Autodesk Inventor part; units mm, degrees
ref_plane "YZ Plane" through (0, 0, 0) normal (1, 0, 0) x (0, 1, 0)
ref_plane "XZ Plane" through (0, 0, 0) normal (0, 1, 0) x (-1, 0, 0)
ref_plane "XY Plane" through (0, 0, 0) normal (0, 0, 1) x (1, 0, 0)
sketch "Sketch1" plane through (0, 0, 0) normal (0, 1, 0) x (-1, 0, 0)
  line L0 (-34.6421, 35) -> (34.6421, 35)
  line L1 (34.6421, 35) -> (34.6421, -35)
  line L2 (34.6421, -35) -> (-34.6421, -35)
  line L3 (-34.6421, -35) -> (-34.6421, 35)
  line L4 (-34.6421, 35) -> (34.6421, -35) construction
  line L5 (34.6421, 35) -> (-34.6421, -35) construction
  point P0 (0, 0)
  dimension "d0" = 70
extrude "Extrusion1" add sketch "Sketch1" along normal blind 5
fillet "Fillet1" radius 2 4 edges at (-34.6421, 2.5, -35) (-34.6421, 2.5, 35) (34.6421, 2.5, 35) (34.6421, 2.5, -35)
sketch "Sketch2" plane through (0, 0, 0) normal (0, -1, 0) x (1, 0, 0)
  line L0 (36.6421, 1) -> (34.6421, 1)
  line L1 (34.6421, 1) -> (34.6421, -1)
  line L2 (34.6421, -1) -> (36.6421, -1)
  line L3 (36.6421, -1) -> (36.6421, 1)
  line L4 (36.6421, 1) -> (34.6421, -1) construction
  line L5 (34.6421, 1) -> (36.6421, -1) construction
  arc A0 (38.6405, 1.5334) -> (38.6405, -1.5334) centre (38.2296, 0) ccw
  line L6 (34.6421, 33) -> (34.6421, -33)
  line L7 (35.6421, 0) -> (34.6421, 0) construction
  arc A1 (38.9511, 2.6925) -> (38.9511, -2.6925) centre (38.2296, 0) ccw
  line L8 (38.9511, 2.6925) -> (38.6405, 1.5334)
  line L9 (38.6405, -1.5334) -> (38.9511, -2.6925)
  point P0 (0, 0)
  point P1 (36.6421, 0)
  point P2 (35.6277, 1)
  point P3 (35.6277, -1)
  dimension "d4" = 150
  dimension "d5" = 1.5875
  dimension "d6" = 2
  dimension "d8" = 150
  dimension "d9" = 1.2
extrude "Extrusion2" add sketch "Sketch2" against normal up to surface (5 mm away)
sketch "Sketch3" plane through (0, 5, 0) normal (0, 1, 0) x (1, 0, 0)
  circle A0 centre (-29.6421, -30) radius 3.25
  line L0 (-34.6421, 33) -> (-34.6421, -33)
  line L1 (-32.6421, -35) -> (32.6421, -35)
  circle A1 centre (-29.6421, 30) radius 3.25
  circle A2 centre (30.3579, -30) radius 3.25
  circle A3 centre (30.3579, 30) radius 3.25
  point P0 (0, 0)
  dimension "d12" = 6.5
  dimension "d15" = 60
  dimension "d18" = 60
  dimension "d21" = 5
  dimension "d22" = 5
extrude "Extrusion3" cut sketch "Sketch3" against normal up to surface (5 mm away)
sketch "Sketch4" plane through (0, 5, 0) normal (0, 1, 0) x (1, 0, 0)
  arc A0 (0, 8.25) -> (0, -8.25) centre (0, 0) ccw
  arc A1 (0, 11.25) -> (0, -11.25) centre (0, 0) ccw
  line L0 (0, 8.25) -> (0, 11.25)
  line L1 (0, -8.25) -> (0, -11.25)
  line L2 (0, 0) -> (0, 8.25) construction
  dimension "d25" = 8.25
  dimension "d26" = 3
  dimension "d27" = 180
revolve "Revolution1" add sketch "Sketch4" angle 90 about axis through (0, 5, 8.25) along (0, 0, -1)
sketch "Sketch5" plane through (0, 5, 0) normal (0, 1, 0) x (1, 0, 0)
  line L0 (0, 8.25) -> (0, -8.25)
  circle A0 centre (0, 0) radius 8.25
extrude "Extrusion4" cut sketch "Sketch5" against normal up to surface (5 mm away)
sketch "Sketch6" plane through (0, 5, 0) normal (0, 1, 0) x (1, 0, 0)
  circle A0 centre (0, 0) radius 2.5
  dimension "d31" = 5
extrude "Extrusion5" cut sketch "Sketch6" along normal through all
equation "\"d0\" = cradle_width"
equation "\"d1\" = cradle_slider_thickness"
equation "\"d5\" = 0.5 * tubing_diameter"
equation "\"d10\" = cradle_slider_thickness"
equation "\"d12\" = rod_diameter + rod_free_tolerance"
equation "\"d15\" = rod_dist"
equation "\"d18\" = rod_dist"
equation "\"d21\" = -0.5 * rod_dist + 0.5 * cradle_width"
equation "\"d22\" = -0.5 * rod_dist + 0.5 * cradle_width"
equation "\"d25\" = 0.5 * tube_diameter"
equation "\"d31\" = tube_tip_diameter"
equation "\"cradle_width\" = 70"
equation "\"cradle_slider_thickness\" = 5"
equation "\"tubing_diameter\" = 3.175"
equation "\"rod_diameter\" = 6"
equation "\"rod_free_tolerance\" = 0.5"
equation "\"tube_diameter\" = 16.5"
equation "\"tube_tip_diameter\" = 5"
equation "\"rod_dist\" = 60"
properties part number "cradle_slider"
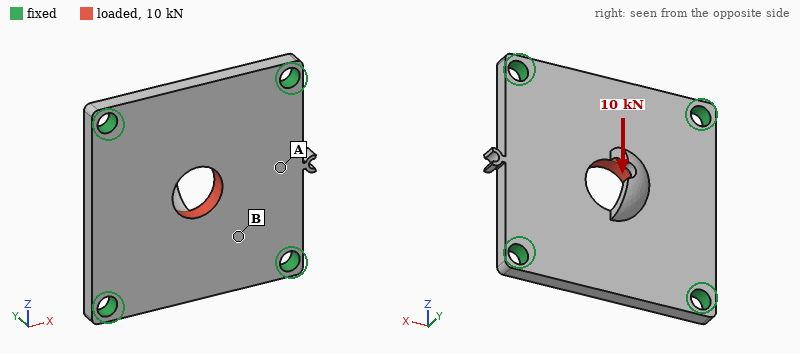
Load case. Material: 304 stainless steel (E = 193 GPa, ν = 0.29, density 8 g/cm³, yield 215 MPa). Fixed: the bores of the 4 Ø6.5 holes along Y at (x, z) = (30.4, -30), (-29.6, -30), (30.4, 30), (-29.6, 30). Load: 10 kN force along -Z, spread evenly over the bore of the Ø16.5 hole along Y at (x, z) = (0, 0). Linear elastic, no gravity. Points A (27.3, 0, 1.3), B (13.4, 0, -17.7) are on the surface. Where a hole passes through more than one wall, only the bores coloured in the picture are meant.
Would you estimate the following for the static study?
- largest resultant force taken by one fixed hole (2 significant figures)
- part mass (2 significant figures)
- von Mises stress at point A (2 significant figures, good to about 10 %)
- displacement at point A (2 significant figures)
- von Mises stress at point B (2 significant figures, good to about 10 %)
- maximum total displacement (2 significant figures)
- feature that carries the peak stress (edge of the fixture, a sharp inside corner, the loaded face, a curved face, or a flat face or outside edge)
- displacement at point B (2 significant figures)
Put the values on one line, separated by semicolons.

2.9 kN; 190 g; 12 MPa; 2.6 µm; 29 MPa; 7.8 µm; edge of the fixture; 4.6 µm
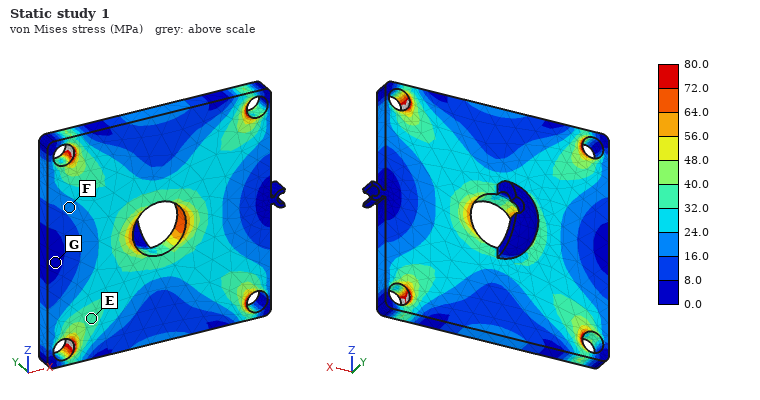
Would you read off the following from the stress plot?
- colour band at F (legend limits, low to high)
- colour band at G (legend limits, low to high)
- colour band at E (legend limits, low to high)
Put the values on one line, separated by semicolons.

16.0 to 24.0 MPa; 0.0 to 8.0 MPa; 32.0 to 40.0 MPa
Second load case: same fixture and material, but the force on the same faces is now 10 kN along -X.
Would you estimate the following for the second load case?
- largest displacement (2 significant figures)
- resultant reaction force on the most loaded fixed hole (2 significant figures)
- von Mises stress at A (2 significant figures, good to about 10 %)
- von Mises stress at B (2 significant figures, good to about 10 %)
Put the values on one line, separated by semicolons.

7.9 µm; 2.9 kN; 9.4 MPa; 30 MPa
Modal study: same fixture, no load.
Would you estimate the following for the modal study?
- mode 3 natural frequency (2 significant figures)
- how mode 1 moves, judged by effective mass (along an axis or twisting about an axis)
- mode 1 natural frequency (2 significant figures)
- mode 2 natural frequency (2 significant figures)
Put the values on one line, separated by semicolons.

8000 Hz; along Y; 4800 Hz; 8000 Hz
